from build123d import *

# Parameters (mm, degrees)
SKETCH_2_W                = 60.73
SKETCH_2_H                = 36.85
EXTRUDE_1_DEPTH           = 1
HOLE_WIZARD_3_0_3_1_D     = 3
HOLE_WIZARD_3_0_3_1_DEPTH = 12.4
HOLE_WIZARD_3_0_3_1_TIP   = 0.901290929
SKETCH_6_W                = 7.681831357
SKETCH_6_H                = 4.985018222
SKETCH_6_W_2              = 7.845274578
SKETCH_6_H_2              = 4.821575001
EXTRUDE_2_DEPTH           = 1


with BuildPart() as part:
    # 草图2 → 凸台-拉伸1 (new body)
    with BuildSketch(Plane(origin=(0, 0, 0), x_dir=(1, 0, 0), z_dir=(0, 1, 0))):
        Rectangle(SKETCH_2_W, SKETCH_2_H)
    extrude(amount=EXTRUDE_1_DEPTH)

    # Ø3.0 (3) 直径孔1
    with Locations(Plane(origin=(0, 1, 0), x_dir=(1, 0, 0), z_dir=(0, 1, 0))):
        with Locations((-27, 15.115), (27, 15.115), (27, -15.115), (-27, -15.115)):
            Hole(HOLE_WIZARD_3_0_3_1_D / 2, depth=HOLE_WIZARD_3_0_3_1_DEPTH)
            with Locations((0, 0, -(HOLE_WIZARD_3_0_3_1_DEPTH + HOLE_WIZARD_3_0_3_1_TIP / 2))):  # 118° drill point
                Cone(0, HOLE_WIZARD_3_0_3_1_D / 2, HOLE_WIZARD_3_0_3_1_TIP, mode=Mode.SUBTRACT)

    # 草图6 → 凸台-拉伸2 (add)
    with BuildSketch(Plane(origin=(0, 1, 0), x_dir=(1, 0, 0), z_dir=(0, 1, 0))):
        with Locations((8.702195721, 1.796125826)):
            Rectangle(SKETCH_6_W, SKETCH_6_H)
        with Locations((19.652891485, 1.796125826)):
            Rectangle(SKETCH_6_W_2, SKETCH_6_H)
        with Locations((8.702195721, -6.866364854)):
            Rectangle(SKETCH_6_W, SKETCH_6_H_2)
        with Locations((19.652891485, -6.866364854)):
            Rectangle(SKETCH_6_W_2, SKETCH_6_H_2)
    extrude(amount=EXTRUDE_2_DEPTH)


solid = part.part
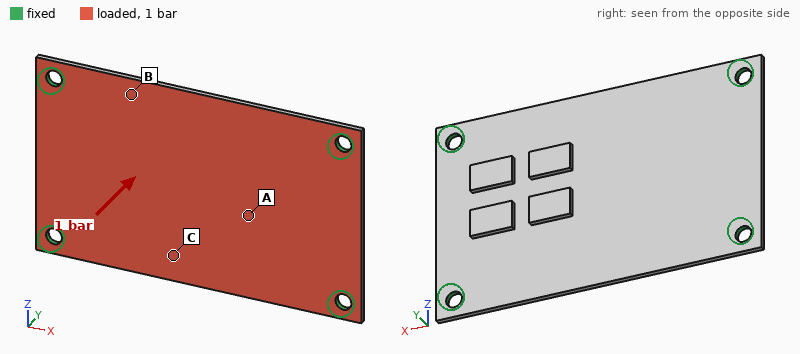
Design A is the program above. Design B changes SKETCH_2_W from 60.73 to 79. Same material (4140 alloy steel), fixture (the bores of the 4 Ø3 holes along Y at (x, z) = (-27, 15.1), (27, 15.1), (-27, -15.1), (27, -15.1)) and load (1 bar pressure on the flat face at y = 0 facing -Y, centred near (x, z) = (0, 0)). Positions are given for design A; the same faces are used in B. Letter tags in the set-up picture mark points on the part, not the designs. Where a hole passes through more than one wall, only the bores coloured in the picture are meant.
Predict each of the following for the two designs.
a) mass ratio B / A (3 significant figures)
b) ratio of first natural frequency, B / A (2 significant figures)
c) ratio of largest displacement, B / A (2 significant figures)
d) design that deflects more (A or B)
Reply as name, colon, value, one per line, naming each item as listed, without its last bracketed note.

mass ratio B / A: 1.29
ratio of first natural frequency, B / A: 1.0
ratio of largest displacement, B / A: 0.92
design that deflects more: A
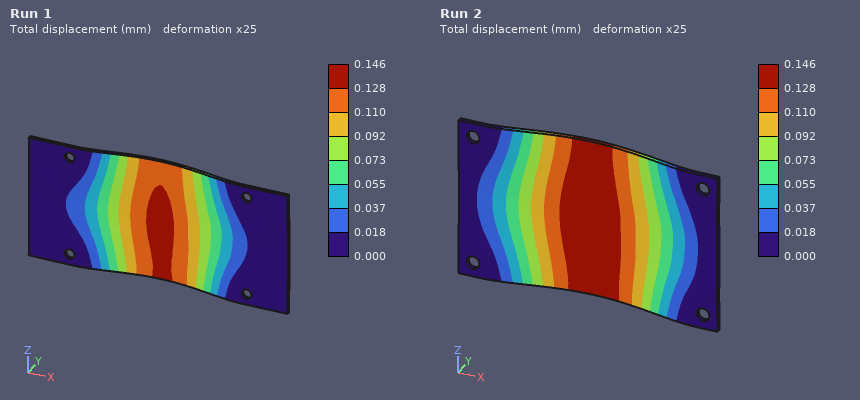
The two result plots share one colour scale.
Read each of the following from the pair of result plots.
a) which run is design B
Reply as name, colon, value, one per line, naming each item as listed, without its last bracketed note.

which run is design B: Run 1
